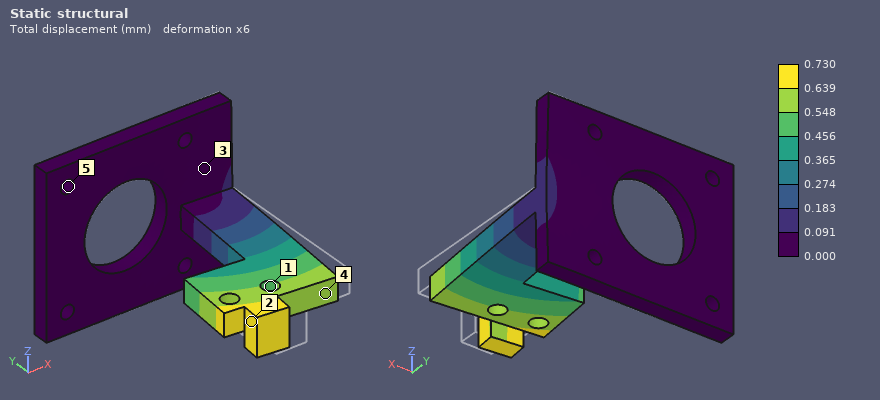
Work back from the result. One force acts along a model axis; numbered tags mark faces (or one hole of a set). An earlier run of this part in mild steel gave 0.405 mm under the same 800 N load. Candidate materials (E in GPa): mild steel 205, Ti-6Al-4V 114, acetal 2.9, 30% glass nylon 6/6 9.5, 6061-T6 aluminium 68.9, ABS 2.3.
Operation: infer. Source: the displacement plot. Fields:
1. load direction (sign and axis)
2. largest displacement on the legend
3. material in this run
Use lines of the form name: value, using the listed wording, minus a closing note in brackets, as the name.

load direction: -X
largest displacement on the legend: 0.730 mm
material in this run: Ti-6Al-4V
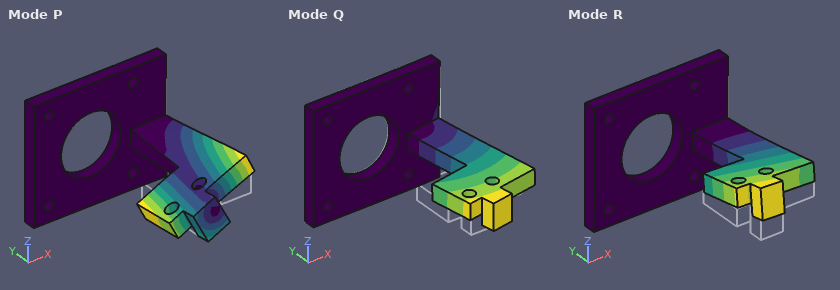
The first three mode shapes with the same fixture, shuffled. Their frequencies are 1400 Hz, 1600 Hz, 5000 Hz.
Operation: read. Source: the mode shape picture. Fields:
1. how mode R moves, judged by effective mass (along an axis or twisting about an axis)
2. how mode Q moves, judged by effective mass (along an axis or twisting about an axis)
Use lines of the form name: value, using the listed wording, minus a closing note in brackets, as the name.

how mode R moves, judged by effective mass: along Z
how mode Q moves, judged by effective mass: along X
